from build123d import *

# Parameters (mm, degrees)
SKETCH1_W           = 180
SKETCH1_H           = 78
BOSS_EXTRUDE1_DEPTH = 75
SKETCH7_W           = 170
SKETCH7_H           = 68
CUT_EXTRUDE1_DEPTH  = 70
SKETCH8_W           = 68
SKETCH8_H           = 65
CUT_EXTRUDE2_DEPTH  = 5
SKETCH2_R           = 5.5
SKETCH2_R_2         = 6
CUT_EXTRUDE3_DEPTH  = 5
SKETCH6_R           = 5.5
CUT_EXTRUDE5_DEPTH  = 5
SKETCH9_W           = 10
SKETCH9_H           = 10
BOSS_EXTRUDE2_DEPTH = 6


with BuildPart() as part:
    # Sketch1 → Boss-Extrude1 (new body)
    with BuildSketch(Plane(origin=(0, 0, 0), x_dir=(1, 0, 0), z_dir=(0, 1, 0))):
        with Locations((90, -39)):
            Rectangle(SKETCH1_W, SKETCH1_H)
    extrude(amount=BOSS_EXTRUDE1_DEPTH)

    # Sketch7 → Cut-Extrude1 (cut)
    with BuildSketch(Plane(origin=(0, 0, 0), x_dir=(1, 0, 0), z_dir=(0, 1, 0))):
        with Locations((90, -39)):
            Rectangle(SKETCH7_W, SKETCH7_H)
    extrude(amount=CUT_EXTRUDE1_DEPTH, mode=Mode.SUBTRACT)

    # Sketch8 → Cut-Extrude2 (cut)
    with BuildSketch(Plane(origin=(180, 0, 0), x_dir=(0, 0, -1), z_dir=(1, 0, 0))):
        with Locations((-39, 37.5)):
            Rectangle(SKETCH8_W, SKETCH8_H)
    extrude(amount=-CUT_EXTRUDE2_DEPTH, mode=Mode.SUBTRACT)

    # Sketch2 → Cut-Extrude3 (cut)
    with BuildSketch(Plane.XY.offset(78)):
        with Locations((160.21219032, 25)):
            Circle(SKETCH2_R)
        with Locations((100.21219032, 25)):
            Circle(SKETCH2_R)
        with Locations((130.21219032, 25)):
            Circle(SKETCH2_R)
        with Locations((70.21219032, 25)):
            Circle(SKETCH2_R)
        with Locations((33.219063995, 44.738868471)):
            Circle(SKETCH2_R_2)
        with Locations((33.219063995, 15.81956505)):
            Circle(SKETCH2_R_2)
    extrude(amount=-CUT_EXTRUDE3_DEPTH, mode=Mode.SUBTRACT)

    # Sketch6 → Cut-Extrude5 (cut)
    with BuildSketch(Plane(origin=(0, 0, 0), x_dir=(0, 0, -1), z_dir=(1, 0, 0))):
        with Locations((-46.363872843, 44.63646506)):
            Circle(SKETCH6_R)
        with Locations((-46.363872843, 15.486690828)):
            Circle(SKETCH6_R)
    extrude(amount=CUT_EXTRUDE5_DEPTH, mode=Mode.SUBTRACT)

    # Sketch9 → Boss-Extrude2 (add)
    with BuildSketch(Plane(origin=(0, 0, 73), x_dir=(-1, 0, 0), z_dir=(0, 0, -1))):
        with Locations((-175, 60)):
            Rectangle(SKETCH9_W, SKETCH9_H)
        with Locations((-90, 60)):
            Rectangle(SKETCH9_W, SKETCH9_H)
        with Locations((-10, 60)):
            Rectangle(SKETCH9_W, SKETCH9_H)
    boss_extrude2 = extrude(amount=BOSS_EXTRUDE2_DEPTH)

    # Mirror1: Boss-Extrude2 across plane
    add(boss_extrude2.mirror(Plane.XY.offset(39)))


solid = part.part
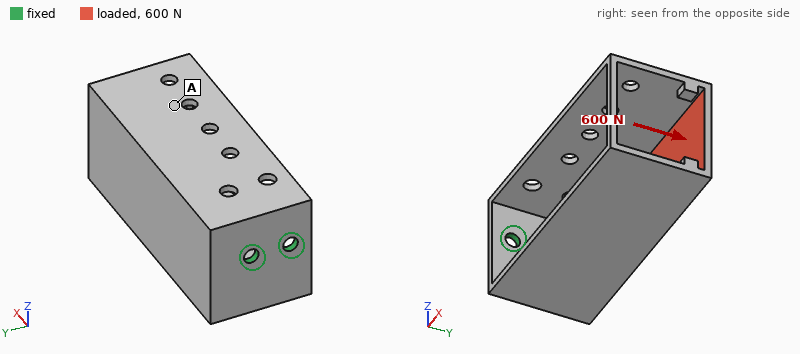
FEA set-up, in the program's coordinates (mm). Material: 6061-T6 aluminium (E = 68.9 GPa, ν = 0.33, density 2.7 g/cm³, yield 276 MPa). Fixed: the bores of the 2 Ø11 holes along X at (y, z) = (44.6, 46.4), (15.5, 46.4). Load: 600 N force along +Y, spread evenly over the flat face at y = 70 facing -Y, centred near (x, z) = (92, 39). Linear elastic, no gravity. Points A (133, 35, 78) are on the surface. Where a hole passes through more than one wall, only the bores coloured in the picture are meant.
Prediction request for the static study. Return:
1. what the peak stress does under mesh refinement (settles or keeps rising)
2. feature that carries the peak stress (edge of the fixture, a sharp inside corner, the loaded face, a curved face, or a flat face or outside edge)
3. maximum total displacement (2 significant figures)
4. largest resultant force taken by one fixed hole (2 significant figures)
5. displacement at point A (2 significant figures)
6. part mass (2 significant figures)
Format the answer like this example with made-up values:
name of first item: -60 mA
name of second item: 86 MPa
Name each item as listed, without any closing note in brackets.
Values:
what the peak stress does under mesh refinement: keeps rising
feature that carries the peak stress: edge of the fixture
maximum total displacement: 0.69 mm
largest resultant force taken by one fixed hole: 1.2 kN
displacement at point A: 0.41 mm
part mass: 600 g
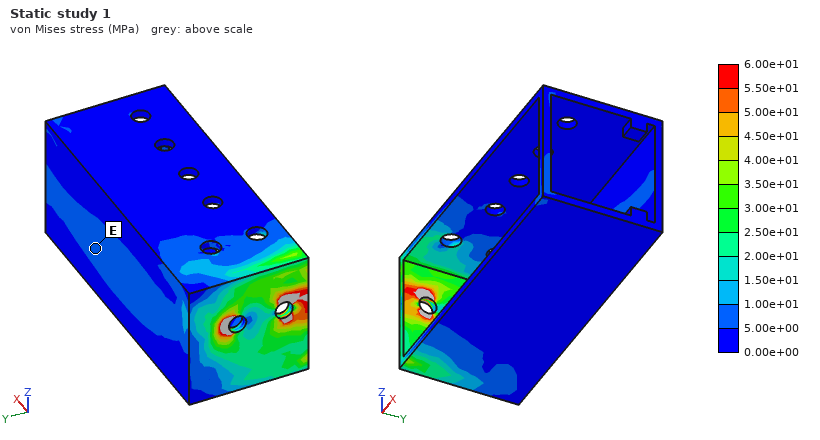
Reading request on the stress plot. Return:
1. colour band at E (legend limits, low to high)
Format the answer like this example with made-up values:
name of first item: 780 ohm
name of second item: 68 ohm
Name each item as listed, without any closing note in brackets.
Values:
colour band at E: 5.00e+00 to 1.00e+01 MPa
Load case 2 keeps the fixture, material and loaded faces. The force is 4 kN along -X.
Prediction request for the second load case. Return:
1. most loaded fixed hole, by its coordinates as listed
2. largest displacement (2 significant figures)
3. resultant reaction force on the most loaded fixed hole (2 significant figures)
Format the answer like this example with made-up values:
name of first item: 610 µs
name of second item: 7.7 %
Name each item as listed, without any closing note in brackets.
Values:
most loaded fixed hole, by its coordinates as listed: (44.6, 46.4)
largest displacement: 1.5 mm
resultant reaction force on the most loaded fixed hole: 5.4 kN
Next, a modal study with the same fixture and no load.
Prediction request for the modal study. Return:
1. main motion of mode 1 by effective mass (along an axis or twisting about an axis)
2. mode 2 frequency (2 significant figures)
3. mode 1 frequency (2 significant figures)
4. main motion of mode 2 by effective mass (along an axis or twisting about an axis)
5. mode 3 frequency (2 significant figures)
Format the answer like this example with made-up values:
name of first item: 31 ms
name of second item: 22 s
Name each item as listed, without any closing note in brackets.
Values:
main motion of mode 1 by effective mass: along Z
mode 2 frequency: 260 Hz
mode 1 frequency: 160 Hz
main motion of mode 2 by effective mass: along Y
mode 3 frequency: 600 Hz
